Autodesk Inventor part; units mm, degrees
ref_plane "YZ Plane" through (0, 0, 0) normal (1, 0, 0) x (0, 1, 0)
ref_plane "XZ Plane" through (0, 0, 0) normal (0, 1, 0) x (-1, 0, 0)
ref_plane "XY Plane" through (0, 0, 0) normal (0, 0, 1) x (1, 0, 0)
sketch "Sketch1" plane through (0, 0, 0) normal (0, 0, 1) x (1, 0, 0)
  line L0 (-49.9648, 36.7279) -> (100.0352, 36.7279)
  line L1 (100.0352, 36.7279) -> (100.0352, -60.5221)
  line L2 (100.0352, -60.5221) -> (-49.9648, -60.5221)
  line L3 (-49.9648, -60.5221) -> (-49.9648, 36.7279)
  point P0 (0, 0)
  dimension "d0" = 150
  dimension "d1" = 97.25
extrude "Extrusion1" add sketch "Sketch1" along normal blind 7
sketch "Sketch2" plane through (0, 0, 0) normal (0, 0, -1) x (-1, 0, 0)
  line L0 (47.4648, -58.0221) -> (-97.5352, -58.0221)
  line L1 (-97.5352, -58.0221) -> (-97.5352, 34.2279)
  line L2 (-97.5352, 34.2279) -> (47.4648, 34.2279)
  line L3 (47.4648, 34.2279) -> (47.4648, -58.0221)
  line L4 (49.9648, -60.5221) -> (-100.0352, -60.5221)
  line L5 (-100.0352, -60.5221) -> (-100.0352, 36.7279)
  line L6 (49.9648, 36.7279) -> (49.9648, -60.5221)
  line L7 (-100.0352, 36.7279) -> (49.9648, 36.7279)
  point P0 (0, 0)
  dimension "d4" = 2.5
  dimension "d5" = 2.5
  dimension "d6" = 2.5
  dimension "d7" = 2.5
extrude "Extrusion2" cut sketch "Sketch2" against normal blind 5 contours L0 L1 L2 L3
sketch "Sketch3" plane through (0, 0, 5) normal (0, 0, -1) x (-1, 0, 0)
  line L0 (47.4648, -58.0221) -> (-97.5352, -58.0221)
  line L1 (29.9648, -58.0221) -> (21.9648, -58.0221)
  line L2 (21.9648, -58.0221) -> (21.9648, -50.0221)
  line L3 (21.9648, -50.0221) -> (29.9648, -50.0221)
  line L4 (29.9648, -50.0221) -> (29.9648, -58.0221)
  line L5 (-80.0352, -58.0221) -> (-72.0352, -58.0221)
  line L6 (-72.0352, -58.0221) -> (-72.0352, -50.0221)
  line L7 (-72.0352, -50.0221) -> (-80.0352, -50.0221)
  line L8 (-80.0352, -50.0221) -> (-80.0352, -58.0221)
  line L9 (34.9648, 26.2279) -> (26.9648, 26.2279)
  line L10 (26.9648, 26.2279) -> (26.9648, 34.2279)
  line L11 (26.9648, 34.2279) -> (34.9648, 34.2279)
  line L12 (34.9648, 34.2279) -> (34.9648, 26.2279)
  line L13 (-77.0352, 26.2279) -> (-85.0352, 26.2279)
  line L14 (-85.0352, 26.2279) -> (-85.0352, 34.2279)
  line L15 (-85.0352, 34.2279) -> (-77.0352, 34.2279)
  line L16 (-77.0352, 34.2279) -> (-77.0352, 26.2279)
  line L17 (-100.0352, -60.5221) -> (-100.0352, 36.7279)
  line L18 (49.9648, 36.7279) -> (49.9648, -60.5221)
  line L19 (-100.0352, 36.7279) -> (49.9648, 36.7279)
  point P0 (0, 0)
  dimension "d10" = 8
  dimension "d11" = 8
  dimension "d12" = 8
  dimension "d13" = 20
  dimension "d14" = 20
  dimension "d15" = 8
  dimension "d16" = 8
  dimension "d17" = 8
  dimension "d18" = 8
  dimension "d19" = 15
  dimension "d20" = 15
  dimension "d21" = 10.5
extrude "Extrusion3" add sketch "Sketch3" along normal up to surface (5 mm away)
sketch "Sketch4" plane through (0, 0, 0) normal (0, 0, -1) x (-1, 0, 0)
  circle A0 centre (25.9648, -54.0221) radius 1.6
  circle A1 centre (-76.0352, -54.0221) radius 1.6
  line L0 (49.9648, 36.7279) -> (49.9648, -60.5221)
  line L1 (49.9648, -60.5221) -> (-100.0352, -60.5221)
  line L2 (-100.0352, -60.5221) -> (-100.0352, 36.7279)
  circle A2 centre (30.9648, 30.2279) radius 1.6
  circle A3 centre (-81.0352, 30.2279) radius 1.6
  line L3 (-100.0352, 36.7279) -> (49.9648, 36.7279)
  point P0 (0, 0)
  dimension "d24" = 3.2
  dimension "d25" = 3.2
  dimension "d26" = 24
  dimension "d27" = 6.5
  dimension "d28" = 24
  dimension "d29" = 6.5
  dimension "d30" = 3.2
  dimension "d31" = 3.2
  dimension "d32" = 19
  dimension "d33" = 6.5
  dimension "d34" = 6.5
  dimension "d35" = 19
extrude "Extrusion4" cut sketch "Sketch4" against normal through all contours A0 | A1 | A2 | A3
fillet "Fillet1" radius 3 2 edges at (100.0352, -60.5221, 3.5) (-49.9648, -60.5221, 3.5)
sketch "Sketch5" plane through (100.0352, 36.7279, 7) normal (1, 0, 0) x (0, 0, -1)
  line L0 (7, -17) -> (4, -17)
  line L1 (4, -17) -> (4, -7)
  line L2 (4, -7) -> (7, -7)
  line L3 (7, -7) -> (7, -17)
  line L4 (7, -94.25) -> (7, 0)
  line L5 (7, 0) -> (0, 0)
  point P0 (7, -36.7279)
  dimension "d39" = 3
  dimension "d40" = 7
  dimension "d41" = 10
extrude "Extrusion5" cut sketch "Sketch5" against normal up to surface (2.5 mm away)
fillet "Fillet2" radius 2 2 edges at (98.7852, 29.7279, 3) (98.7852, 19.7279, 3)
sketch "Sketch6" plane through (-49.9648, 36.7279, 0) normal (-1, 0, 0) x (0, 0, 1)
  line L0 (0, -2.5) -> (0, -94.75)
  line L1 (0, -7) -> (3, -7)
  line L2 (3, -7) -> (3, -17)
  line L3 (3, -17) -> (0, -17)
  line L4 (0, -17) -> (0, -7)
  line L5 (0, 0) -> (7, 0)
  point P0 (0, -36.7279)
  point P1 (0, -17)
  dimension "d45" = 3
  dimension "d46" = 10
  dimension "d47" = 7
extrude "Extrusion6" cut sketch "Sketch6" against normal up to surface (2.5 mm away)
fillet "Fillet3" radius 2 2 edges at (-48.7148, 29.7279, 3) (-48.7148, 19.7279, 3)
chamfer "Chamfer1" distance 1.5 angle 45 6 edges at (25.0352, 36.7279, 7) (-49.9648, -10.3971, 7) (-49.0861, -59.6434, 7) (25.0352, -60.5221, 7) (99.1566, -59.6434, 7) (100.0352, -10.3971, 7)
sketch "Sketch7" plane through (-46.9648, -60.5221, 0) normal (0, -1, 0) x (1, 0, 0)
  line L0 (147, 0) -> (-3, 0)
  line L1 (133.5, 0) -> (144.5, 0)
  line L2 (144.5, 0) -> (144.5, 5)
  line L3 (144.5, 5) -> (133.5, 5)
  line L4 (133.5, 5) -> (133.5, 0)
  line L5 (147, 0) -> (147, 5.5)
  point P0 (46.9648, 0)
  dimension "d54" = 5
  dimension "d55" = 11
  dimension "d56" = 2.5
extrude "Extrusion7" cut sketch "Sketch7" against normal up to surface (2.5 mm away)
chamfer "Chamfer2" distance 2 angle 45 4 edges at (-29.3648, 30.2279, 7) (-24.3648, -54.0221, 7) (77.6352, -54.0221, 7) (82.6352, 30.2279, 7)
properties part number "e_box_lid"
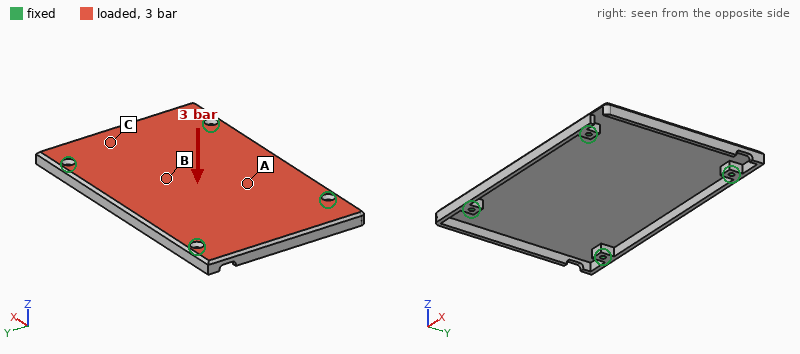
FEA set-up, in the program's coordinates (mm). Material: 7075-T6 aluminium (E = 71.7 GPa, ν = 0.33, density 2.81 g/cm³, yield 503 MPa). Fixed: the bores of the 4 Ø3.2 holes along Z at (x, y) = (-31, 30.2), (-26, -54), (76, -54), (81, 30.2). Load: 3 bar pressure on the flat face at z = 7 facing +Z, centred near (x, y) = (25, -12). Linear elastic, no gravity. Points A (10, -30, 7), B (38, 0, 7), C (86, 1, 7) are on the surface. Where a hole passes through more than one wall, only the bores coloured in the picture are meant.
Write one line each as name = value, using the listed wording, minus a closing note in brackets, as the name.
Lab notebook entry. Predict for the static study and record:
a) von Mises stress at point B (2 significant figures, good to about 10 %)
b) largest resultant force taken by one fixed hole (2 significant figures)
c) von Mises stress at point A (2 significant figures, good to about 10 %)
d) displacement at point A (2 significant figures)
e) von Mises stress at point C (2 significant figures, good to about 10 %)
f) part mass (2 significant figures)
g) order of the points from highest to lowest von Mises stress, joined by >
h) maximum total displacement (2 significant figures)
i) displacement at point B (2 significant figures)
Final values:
von Mises stress at point B = 180 MPa
largest resultant force taken by one fixed hole = 1.6 kN
von Mises stress at point A = 150 MPa
displacement at point A = 1.6 mm
von Mises stress at point C = 100 MPa
part mass = 99 g
order of the points from highest to lowest von Mises stress, joined by > = B > A > C
maximum total displacement = 2.1 mm
displacement at point B = 1.9 mm
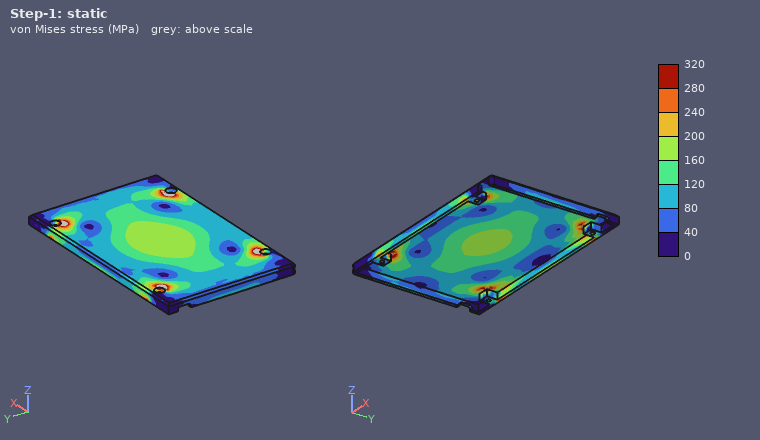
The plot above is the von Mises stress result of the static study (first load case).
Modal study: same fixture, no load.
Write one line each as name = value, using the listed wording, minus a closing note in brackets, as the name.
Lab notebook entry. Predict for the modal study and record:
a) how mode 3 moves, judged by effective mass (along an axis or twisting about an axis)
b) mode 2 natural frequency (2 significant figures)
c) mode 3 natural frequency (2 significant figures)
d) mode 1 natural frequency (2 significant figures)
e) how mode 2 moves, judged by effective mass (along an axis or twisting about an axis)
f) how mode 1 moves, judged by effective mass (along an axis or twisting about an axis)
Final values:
how mode 3 moves, judged by effective mass = along Z
mode 2 natural frequency = 1800 Hz
mode 3 natural frequency = 1900 Hz
mode 1 natural frequency = 990 Hz
how mode 2 moves, judged by effective mass = twisting about Y
how mode 1 moves, judged by effective mass = along Z
